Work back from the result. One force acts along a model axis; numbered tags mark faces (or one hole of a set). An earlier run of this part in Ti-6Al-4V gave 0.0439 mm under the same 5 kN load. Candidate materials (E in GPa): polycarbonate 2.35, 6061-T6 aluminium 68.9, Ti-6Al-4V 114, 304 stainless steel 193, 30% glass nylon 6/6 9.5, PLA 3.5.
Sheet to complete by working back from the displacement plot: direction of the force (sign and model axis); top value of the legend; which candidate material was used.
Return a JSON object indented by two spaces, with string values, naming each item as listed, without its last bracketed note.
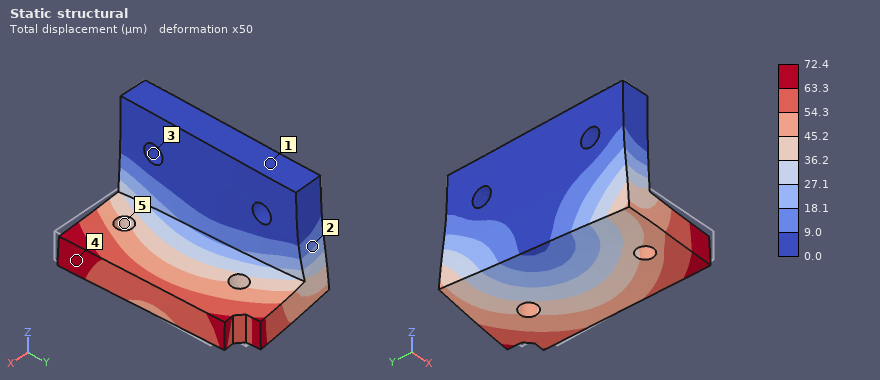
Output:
{
  "direction of the force": "+Y",
  "top value of the legend": "72.4 µm",
  "which candidate material was used": "6061-T6 aluminium"
}
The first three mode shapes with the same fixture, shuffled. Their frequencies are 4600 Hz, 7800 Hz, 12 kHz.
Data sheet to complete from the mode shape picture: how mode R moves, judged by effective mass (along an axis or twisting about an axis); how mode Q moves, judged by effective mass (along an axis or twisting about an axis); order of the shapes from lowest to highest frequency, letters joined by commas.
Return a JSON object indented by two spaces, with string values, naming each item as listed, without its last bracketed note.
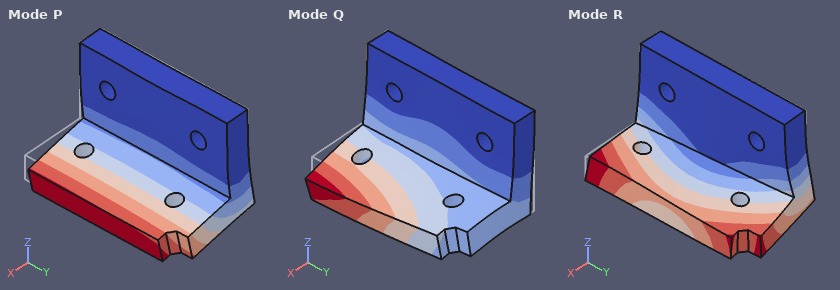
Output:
{
  "how mode R moves, judged by effective mass": "along Y",
  "how mode Q moves, judged by effective mass": "along X",
  "order of the shapes from lowest to highest frequency, letters joined by commas": "P, R, Q"
}
